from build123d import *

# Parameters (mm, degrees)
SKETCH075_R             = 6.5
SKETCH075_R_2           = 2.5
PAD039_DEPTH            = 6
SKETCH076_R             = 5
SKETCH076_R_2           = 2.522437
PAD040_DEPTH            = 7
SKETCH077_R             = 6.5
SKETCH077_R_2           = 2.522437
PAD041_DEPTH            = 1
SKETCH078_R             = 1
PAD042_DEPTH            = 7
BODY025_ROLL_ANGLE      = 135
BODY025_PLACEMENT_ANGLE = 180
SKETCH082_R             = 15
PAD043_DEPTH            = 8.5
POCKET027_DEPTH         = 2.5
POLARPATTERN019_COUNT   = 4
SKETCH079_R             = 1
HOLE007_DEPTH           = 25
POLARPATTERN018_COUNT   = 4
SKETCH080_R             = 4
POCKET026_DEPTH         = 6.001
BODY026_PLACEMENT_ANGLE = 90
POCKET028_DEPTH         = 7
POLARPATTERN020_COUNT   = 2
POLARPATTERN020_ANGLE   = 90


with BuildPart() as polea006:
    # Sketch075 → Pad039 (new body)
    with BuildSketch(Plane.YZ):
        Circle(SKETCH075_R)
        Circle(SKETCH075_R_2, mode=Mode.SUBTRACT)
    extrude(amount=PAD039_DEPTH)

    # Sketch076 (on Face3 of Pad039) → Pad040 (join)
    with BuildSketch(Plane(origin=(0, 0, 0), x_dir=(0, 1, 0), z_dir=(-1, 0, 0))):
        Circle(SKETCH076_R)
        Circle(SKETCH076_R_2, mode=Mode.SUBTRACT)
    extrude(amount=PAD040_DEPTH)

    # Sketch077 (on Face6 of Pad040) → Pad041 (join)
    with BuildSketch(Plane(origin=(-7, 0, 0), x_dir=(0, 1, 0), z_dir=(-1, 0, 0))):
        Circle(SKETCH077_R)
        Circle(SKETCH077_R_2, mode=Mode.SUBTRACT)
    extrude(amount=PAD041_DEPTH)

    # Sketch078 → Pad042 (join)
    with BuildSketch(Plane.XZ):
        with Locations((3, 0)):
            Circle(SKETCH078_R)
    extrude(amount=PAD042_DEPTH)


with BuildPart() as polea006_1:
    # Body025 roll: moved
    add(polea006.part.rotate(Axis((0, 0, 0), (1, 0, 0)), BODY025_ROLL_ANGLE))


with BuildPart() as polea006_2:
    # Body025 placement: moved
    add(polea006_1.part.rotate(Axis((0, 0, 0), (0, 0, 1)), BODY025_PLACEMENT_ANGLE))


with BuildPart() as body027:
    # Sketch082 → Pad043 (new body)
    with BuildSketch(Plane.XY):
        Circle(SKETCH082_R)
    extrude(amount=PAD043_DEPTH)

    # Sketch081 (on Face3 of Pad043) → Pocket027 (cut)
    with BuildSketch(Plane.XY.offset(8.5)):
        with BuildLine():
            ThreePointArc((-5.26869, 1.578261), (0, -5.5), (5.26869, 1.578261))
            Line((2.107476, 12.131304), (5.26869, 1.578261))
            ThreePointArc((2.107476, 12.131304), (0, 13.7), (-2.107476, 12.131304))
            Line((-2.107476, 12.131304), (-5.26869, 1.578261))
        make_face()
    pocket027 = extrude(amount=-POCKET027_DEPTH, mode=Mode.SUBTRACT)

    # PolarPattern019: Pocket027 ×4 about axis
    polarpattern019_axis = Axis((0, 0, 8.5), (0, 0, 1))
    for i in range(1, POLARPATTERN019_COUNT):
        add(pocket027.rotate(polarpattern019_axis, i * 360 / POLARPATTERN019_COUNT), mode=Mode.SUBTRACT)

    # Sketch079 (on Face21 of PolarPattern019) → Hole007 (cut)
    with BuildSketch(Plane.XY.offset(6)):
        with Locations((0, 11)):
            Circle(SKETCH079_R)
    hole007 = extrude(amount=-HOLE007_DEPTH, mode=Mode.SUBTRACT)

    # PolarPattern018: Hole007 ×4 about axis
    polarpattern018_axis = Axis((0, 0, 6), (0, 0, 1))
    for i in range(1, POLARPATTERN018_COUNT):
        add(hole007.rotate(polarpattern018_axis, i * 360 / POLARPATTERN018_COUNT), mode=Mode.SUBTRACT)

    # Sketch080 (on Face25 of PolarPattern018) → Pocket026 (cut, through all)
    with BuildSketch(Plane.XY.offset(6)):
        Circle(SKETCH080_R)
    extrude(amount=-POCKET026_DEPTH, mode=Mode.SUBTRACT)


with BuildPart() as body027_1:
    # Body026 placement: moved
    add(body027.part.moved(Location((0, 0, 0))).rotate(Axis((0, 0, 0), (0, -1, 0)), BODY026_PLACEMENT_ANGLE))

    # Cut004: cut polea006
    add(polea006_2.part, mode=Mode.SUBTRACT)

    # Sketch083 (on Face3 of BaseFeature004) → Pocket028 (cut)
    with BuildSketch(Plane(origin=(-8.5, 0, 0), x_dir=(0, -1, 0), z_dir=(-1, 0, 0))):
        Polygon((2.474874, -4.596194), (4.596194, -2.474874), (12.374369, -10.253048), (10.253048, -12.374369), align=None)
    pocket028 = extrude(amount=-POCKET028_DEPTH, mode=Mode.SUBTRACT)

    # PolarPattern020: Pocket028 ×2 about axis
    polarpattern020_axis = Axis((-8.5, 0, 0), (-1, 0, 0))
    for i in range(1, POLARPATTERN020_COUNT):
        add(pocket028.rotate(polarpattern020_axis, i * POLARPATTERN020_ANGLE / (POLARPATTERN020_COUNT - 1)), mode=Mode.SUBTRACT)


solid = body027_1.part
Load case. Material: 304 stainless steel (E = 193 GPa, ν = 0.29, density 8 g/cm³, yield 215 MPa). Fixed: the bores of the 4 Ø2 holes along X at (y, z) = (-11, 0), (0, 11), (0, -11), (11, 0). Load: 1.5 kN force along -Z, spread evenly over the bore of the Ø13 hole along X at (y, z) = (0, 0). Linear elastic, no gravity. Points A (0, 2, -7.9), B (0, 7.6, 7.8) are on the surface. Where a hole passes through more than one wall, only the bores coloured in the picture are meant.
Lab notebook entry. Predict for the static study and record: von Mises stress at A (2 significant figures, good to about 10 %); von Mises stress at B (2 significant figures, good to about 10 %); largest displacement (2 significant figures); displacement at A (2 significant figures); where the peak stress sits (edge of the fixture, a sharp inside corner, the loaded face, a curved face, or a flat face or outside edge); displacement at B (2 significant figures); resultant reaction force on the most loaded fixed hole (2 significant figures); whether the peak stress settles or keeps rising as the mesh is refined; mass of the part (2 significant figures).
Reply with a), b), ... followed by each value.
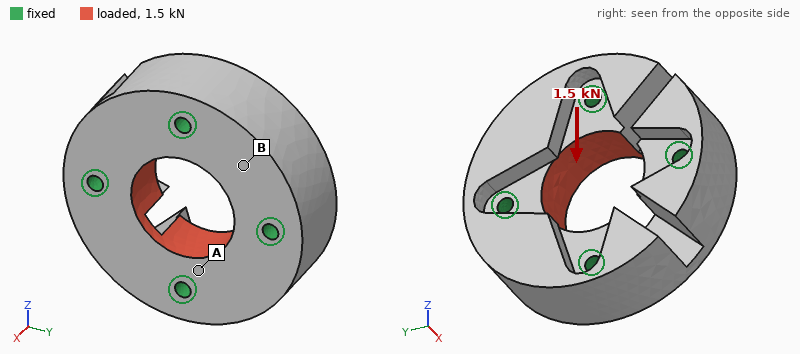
a) 11 MPa
b) 3.9 MPa
c) 0.72 µm
d) 0.22 µm
e) edge of the fixture
f) 0.30 µm
g) 410 N
h) keeps rising
i) 32 g
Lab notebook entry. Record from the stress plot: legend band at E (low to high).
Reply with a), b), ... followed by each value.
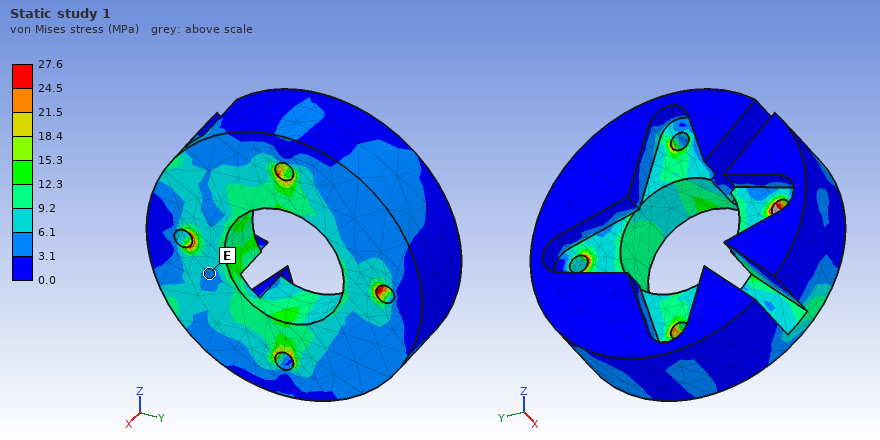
a) 3.1 to 6.1 MPa
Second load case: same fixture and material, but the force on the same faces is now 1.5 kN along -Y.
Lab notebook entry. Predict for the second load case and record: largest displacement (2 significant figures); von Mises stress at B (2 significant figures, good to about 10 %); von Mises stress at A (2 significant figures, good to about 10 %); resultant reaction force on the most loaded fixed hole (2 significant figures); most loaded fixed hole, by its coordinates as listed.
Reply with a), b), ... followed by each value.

a) 0.65 µm
b) 4.3 MPa
c) 7.2 MPa
d) 440 N
e) (11, 0)
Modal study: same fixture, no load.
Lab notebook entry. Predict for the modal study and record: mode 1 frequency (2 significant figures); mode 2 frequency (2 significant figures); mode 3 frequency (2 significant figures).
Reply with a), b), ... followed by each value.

a) 41 kHz
b) 45 kHz
c) 46 kHz
